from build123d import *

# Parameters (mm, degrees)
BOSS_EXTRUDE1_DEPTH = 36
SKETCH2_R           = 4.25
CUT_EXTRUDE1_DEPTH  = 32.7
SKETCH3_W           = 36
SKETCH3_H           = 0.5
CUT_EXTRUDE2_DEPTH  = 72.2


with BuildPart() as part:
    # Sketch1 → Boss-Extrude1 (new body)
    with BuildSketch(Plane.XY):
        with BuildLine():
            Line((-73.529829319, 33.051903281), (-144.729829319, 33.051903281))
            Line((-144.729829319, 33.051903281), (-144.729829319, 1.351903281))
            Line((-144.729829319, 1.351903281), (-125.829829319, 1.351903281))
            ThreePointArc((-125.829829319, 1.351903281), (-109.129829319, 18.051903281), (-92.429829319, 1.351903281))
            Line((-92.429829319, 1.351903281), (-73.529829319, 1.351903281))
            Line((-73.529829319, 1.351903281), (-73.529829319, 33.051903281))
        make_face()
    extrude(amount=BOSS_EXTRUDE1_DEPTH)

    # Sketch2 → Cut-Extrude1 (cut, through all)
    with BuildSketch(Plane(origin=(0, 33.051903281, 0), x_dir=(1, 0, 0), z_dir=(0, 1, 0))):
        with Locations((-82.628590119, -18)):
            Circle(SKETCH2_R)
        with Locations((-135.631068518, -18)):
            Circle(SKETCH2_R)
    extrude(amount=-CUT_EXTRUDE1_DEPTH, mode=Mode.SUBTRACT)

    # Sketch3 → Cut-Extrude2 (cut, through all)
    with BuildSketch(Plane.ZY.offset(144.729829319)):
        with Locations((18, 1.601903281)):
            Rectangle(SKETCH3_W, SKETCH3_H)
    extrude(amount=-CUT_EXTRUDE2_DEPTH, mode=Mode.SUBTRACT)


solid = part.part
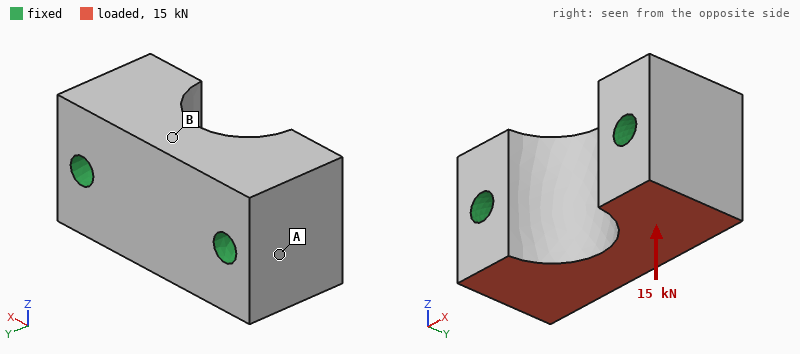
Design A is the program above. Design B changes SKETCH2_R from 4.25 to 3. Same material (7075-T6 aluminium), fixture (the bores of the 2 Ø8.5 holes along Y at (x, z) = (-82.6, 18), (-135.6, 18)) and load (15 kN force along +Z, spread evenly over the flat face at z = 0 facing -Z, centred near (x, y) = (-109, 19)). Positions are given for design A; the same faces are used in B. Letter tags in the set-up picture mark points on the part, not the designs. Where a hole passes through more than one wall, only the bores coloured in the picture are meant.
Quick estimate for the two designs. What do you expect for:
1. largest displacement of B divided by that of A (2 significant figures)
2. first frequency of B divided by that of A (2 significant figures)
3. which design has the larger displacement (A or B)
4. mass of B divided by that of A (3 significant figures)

1.2
0.88
B
1.03
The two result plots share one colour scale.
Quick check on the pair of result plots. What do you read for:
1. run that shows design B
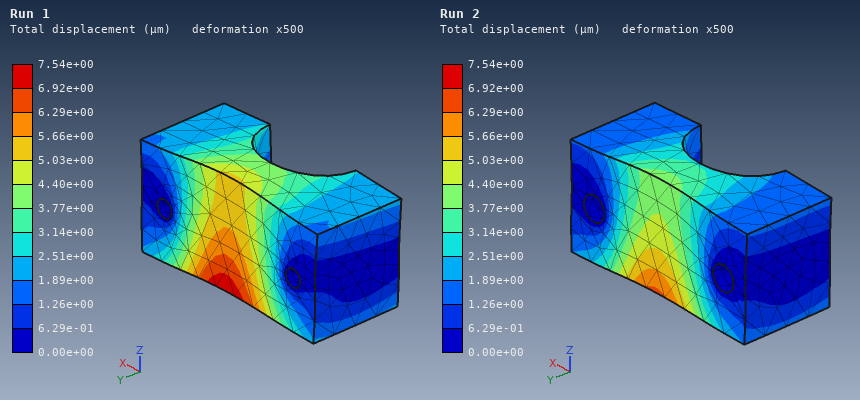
Run 1
